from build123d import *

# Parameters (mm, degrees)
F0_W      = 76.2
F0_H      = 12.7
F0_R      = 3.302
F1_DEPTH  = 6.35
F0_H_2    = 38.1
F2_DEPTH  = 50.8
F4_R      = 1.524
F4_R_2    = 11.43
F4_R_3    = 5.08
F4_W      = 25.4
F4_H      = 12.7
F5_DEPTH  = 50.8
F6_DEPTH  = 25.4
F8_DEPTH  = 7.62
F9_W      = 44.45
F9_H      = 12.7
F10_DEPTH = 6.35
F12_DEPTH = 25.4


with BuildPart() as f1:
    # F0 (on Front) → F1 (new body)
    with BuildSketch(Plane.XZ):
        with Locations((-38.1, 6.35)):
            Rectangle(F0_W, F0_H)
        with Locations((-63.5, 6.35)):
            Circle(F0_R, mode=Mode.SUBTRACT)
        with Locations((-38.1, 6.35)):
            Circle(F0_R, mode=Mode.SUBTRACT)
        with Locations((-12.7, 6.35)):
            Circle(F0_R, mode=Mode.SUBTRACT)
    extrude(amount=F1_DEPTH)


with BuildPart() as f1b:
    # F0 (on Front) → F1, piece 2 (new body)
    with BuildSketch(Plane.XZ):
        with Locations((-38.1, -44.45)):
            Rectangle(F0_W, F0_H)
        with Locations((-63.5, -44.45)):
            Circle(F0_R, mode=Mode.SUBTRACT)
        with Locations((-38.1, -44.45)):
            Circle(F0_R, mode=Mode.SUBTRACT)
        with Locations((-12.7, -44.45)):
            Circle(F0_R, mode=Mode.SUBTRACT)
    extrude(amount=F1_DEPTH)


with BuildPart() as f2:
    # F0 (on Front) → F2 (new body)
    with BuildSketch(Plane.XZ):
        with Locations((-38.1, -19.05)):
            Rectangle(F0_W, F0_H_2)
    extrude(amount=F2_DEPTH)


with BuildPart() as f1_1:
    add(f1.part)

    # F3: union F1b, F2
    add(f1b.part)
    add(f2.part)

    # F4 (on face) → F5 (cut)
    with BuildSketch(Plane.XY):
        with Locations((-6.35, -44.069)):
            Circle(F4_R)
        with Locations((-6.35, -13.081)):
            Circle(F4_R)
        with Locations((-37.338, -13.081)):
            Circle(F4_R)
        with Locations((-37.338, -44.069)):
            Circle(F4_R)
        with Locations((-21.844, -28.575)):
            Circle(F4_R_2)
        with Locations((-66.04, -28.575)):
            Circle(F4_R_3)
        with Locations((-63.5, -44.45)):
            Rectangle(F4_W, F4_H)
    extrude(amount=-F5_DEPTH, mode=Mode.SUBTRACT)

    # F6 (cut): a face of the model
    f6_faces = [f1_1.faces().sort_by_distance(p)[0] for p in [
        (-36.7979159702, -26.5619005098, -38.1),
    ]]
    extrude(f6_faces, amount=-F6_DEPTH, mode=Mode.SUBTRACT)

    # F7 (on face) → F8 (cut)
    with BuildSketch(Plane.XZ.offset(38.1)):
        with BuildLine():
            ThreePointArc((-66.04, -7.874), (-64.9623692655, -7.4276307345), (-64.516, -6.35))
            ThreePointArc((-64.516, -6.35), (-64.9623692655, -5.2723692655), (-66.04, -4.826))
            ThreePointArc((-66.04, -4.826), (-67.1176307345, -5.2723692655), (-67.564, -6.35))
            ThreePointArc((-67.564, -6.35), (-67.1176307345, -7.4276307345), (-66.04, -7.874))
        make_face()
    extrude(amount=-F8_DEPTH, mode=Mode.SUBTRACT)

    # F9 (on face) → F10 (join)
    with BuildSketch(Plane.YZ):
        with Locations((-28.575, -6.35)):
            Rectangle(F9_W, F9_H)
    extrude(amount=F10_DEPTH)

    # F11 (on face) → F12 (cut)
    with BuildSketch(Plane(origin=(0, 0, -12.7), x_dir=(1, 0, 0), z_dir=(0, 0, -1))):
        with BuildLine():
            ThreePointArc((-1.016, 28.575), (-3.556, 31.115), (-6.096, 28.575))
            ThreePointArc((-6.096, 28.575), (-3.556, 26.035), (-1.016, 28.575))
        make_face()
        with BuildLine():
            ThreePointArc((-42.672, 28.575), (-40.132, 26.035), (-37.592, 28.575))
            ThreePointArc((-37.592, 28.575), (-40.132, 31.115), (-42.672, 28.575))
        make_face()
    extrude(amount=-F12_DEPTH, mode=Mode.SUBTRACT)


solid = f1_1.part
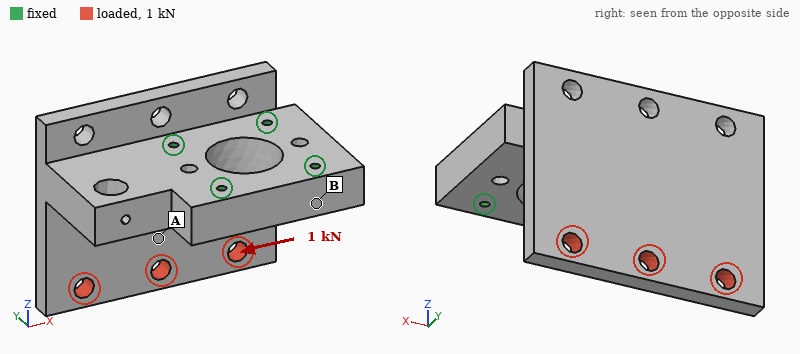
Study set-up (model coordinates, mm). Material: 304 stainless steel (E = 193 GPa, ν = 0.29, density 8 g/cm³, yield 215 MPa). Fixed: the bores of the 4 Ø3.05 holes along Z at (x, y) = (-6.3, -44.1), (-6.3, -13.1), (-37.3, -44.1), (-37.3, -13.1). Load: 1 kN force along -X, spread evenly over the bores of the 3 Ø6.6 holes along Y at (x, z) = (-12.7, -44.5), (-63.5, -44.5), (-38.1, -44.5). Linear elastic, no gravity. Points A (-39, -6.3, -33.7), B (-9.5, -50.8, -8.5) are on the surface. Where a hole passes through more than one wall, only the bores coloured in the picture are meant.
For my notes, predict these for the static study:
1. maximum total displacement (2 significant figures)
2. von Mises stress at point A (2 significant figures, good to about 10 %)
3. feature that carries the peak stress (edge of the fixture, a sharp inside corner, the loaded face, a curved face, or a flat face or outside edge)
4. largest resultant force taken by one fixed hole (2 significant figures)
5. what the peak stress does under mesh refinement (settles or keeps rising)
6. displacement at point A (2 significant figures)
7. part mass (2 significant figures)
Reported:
8.6 µm
6.4 MPa
edge of the fixture
1.2 kN
keeps rising
3.9 µm
520 g
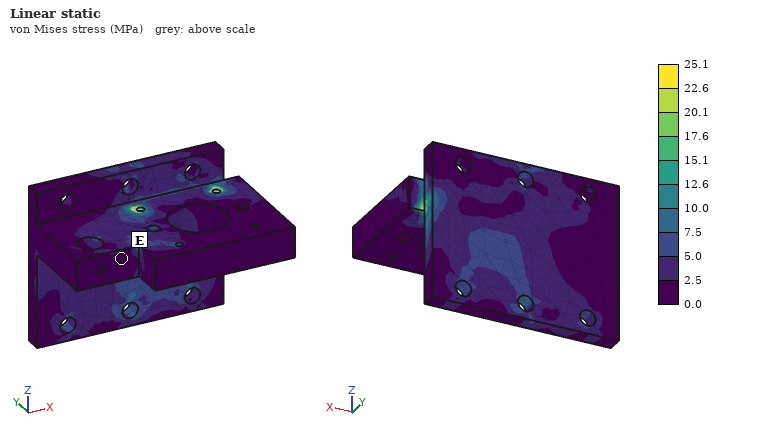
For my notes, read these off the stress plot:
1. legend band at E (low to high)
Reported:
0.0 to 2.5 MPa
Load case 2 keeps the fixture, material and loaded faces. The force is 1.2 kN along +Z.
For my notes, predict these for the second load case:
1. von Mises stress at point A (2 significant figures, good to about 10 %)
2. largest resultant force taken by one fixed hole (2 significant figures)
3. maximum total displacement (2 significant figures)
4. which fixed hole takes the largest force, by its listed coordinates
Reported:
3.5 MPa
1.2 kN
6.0 µm
(-37.3, -13.1)
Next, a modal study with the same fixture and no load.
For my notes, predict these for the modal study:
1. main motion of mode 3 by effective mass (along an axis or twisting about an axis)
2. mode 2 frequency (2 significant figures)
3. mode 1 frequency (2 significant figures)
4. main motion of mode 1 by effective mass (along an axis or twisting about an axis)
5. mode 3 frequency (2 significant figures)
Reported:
along Z
4400 Hz
2800 Hz
along Y
5400 Hz
